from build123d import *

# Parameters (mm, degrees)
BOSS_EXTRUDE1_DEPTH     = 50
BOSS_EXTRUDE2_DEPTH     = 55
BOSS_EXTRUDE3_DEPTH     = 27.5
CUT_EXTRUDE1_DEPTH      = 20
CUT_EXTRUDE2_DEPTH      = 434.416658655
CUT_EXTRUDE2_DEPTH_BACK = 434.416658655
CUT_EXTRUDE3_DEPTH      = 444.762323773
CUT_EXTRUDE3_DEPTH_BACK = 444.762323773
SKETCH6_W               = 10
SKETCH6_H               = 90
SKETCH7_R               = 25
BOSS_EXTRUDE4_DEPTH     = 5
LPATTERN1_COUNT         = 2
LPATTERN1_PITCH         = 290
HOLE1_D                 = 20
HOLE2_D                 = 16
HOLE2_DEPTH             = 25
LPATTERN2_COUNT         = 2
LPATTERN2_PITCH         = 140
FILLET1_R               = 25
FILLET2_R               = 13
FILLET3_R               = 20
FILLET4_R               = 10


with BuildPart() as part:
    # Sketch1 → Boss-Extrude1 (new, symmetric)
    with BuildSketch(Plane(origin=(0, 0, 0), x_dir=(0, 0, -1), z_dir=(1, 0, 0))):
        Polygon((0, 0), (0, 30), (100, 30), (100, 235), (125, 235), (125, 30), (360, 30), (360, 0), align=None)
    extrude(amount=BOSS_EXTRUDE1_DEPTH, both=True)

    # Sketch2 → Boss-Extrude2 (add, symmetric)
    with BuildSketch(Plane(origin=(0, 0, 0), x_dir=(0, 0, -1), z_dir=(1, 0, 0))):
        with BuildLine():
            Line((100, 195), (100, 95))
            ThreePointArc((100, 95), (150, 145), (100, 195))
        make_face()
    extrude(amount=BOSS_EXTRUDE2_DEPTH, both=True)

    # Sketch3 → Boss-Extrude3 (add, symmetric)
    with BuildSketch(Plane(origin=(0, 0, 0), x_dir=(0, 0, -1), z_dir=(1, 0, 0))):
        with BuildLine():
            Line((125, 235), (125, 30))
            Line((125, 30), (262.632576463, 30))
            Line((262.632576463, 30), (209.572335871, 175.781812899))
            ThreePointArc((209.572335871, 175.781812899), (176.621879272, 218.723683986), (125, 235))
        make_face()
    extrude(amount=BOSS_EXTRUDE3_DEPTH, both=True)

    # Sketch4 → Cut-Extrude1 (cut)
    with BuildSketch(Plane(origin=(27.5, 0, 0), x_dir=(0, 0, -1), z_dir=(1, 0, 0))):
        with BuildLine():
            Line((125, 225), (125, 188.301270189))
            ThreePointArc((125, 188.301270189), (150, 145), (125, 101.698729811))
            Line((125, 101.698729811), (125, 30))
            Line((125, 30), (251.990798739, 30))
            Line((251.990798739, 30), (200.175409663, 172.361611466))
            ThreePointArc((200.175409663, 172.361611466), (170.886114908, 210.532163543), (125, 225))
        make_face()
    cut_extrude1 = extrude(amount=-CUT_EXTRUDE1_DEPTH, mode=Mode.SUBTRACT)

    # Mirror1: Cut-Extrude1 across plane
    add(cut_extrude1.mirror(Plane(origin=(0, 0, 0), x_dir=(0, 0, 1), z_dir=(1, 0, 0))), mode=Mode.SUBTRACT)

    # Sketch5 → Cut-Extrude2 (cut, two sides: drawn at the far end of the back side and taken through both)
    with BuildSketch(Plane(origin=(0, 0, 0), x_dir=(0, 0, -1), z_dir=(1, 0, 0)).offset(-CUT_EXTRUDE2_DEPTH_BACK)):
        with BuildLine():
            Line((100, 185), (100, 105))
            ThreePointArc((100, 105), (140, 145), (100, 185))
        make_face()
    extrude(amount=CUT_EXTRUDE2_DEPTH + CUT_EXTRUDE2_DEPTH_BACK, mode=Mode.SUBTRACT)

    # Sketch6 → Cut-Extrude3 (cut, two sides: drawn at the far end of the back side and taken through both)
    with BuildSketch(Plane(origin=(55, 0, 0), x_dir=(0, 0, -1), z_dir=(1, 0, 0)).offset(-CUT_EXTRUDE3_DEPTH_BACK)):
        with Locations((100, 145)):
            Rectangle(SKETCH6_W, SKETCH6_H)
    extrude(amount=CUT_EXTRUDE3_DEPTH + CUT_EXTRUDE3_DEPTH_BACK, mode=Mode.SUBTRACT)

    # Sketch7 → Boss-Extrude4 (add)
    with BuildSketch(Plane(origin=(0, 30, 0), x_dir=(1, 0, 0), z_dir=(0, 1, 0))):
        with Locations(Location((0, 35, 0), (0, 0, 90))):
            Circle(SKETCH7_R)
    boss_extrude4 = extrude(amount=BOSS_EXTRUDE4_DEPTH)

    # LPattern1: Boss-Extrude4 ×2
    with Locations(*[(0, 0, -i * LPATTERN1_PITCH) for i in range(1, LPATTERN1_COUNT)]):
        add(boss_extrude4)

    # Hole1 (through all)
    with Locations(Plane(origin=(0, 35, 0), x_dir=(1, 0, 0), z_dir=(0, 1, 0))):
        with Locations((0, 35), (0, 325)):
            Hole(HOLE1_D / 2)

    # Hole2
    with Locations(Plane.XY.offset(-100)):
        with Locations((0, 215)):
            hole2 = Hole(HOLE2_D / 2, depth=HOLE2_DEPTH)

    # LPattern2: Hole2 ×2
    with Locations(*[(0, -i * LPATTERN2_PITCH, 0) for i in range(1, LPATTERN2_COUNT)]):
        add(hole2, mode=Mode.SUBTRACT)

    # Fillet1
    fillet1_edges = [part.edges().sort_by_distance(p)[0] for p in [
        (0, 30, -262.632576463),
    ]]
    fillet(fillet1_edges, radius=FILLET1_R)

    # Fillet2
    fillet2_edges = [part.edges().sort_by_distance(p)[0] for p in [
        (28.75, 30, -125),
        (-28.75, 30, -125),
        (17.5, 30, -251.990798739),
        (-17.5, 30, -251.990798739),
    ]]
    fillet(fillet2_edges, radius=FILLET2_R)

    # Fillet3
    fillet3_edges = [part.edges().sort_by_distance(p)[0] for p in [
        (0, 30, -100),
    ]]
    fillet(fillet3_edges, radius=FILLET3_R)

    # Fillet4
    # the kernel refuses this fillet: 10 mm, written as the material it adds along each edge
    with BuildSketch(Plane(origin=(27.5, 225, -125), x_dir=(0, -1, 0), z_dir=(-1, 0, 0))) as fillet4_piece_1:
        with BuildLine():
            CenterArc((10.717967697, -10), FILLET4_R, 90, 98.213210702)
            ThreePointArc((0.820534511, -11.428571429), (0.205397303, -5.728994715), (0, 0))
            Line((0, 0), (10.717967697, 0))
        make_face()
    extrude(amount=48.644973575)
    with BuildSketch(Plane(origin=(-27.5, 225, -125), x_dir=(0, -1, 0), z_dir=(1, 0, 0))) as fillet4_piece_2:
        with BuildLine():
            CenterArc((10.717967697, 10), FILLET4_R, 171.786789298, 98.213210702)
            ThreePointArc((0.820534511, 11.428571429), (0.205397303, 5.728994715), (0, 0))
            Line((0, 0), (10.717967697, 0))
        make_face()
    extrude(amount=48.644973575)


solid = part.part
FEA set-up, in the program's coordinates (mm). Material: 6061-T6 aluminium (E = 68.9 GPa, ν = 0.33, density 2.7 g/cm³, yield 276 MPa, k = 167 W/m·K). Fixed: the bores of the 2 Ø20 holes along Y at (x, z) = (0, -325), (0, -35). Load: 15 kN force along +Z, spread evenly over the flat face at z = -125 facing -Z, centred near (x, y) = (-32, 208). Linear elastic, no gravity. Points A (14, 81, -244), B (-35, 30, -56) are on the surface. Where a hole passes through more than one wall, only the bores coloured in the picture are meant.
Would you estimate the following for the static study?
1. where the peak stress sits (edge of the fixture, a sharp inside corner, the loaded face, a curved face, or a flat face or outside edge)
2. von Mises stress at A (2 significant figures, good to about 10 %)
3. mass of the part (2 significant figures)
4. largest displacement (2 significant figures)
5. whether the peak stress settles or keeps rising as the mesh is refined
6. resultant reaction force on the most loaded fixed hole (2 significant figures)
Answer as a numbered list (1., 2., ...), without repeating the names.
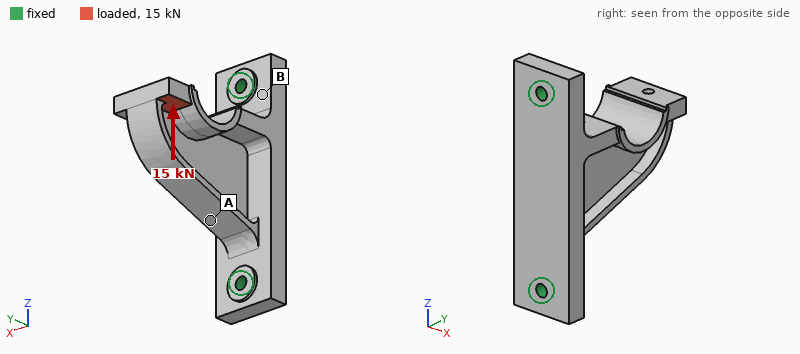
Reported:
1. a sharp inside corner
2. 38 MPa
3. 5.1 kg
4. 0.87 mm
5. keeps rising
6. 15 kN
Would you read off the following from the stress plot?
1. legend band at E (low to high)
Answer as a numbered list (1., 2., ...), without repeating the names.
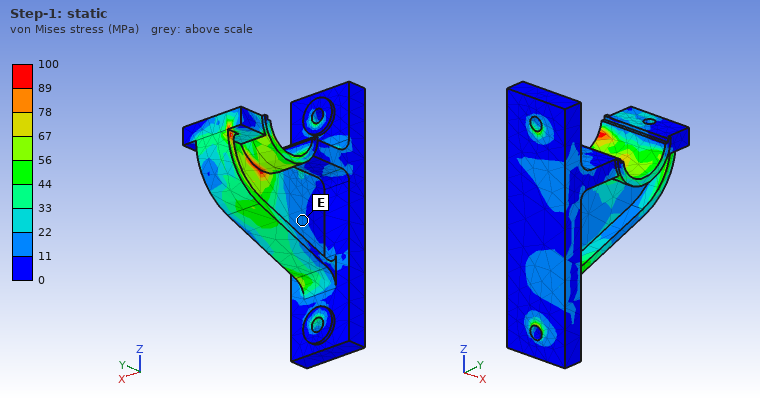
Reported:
1. 11 to 22 MPa
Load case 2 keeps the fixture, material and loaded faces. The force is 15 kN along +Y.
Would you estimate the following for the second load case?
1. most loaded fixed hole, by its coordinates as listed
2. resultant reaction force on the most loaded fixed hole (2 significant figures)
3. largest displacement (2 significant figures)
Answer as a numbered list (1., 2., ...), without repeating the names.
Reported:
1. (0, -35)
2. 11 kN
3. 0.53 mm
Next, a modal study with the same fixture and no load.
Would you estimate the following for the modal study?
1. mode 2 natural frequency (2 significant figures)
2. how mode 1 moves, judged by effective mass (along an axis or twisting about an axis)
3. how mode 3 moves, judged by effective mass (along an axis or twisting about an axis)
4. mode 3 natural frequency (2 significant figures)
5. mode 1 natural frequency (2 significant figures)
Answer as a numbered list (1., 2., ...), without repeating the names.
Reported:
1. 1200 Hz
2. along X
3. along Z
4. 1400 Hz
5. 520 Hz
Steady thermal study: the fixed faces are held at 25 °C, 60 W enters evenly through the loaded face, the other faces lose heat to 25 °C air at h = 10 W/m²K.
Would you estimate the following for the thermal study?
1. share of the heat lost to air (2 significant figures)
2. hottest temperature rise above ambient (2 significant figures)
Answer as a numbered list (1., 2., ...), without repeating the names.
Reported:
1. 28 %
2. 31 K
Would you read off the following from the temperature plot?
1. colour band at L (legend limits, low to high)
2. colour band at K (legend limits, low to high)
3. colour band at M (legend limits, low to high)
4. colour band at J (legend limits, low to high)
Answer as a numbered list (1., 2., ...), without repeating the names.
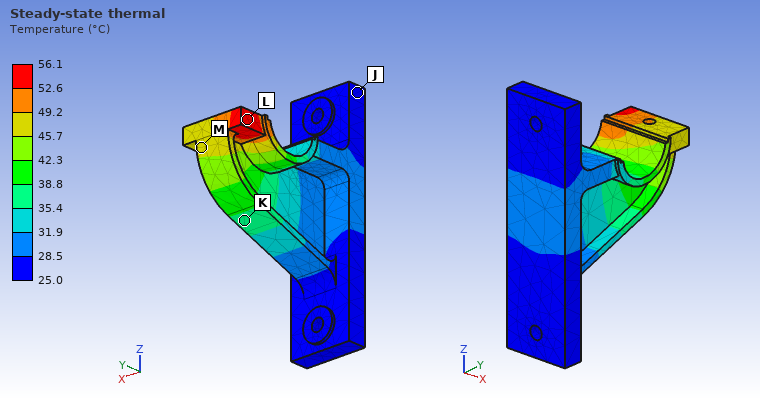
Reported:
1. 52.6 to 56.1 °C
2. 35.4 to 38.8 °C
3. 45.7 to 49.2 °C
4. 25.0 to 28.5 °C
